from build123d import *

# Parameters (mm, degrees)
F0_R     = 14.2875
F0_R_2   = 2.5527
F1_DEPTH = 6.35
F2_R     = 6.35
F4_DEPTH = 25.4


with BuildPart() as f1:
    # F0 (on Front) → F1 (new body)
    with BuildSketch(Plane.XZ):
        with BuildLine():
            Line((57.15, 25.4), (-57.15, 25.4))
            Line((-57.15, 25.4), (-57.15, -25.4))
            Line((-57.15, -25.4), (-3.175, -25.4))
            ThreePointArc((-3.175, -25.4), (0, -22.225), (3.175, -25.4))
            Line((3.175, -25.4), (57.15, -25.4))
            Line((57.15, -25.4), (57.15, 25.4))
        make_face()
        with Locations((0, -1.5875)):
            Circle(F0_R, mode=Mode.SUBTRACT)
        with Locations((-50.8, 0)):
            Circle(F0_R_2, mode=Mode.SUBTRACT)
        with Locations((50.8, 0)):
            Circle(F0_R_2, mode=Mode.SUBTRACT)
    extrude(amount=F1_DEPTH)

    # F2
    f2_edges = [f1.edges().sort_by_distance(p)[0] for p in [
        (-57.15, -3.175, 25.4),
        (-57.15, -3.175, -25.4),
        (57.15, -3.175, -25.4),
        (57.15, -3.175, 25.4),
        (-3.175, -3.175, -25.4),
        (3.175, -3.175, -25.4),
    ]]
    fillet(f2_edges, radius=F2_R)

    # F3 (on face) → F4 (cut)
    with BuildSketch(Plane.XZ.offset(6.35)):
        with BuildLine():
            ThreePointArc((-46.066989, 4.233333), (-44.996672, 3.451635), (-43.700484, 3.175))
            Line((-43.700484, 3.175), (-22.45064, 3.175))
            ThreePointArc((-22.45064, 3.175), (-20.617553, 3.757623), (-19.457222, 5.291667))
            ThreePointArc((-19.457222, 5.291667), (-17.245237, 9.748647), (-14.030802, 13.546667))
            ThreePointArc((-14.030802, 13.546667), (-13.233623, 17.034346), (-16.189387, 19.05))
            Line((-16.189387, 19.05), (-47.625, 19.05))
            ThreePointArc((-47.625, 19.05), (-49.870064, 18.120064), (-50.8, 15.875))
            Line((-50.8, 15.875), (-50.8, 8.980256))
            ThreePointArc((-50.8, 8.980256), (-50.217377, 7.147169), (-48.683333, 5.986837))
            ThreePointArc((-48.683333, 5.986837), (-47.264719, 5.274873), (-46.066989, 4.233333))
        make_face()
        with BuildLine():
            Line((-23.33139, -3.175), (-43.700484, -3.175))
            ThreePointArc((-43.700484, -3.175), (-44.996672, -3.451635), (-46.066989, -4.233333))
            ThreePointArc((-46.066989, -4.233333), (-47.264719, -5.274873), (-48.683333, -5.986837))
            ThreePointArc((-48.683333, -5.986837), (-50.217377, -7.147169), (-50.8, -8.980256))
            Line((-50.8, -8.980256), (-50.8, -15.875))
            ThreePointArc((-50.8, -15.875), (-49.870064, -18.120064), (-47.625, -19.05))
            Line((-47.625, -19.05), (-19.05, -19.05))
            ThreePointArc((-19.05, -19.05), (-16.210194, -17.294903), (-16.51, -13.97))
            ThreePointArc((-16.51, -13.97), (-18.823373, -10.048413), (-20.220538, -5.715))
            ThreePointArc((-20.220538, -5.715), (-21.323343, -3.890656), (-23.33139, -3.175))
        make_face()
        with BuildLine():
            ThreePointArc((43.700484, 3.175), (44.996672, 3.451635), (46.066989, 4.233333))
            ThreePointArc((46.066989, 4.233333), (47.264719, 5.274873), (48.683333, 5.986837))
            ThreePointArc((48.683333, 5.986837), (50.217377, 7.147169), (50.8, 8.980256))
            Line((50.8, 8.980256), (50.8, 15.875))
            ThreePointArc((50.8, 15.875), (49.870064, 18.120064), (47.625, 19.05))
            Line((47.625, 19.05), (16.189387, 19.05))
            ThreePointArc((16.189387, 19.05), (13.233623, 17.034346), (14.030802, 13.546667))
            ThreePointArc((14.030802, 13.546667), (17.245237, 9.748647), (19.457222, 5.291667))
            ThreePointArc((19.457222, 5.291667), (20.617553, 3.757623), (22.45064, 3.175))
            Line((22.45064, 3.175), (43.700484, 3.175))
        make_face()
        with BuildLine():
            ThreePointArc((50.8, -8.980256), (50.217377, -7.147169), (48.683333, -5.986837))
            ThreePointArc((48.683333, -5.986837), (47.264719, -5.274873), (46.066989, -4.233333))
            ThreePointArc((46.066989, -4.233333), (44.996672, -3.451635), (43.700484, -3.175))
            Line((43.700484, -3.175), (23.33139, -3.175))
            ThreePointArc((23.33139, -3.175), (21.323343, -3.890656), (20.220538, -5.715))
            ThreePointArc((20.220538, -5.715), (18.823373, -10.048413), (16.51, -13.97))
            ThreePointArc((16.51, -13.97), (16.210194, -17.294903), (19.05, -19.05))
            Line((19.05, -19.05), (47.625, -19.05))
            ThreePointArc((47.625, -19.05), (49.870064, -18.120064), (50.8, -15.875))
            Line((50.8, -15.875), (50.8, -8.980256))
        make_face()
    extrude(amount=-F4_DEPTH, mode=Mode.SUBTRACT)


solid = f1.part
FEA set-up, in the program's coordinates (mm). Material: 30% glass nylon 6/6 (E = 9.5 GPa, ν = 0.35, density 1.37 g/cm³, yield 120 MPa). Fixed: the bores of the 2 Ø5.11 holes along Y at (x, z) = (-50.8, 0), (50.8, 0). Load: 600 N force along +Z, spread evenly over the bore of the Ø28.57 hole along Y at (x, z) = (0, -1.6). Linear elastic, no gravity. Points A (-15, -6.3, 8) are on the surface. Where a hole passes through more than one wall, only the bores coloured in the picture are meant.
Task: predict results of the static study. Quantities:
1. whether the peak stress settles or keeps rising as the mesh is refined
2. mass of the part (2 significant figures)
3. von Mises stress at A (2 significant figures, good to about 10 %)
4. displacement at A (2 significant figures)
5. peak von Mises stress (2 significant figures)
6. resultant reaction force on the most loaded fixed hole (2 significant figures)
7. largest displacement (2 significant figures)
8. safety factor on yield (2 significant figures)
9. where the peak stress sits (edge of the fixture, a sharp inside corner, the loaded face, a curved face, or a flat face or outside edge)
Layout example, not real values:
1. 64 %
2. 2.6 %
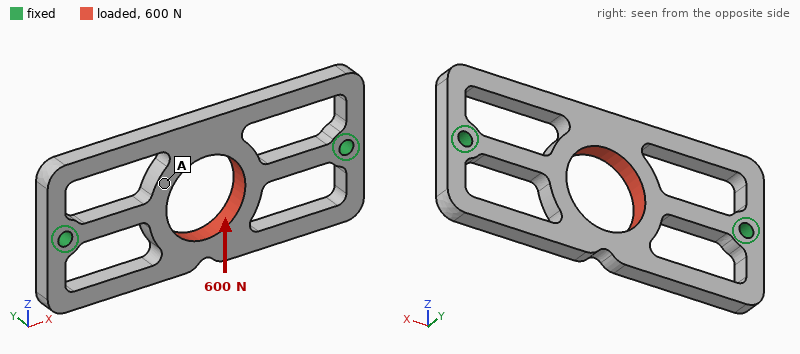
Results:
1. settles
2. 26 g
3. 8.9 MPa
4. 0.33 mm
5. 63 MPa
6. 300 N
7. 0.34 mm
8. 1.9
9. a curved face
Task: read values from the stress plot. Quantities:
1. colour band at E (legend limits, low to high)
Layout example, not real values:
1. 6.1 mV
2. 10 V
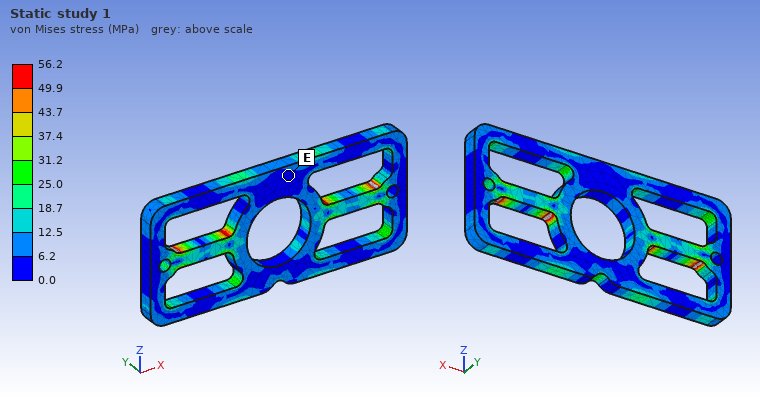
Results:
1. 0.0 to 6.2 MPa
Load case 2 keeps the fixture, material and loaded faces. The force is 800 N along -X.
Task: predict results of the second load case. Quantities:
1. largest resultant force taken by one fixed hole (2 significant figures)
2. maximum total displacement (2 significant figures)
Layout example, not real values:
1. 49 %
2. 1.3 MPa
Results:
1. 400 N
2. 51 µm
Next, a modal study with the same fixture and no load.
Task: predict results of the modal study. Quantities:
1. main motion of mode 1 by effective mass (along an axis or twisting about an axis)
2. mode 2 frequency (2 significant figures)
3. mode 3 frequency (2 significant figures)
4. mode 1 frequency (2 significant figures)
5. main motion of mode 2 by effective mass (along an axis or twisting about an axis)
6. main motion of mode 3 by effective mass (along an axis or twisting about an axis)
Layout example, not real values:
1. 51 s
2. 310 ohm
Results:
1. along Y
2. 1100 Hz
3. 1900 Hz
4. 1000 Hz
5. twisting about X
6. along Z
